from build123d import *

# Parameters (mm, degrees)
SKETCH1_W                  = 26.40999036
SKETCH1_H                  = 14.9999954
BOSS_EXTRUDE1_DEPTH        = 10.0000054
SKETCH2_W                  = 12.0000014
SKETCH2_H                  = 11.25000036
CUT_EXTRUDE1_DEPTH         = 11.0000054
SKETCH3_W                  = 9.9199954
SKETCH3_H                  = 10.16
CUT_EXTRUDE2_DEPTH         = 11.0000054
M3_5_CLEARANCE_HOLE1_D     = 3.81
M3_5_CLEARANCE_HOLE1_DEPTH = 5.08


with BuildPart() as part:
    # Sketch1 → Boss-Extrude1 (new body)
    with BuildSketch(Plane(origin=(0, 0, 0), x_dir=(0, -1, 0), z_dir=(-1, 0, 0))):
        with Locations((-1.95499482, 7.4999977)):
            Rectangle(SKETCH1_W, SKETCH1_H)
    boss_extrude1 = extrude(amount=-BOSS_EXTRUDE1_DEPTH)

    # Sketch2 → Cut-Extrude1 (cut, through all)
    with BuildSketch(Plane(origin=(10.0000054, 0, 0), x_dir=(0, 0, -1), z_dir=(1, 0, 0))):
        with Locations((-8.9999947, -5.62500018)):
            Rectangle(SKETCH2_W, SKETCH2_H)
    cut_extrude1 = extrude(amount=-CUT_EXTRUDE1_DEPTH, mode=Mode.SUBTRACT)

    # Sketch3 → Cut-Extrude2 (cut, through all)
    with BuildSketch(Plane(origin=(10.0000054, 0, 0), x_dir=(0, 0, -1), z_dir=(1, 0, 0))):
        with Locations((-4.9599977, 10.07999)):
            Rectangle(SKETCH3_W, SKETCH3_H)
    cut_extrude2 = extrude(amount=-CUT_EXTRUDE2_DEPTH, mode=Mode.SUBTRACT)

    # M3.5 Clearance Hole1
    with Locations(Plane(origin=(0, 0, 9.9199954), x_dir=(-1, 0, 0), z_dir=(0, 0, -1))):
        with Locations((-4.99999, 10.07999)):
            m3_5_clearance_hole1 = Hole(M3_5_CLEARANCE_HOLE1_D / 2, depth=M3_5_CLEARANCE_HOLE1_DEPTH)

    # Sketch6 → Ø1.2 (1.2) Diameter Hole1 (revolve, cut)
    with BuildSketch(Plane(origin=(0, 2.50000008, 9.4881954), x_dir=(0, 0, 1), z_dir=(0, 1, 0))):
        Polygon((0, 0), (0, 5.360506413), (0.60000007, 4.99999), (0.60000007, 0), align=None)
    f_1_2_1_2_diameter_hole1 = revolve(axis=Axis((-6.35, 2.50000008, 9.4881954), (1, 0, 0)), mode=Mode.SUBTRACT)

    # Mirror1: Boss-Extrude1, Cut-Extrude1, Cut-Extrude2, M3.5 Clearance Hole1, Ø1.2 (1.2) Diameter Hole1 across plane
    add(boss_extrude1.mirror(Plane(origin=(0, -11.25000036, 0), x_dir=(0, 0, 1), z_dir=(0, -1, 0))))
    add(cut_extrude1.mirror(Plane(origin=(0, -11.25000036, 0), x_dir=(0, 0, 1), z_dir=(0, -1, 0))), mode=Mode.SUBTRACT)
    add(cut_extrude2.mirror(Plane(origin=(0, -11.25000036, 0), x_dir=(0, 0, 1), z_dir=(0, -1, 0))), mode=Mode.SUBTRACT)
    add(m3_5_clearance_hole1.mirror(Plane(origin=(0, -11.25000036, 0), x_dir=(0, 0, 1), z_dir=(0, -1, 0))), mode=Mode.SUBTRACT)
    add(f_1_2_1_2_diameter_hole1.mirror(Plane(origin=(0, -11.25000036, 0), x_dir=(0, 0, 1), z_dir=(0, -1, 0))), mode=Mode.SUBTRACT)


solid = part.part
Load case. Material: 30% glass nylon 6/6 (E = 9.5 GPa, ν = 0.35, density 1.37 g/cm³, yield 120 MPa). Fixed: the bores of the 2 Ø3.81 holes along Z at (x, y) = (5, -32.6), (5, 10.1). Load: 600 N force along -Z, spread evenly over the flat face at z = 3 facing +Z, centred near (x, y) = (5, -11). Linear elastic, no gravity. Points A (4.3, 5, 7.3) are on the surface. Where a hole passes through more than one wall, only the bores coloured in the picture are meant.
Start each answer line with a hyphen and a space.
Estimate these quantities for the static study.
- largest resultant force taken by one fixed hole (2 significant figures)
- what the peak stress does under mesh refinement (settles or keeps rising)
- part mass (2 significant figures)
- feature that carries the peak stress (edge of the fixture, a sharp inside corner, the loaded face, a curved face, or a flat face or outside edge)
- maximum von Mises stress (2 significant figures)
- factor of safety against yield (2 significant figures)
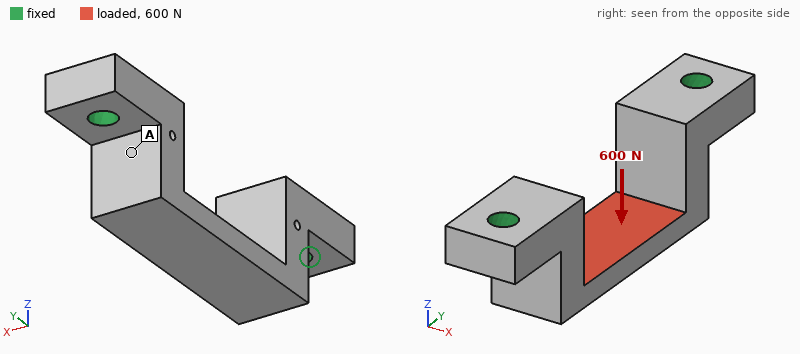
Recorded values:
- 390 N
- settles
- 4.2 g
- a flat face or outside edge
- 61 MPa
- 2.0
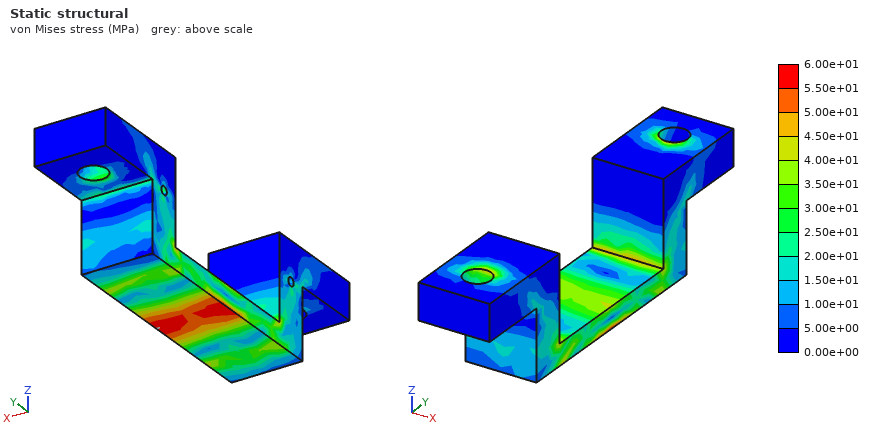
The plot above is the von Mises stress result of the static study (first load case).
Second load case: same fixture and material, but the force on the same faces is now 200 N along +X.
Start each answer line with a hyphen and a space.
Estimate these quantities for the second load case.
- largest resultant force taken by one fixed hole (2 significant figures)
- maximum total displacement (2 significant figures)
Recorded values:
- 100 N
- 99 µm
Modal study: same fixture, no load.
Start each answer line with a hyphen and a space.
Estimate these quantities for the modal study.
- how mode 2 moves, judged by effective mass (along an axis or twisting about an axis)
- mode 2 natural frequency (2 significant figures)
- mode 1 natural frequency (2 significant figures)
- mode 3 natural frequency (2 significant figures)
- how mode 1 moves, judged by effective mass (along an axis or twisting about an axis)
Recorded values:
- along Y
- 6800 Hz
- 5800 Hz
- 9300 Hz
- along X
